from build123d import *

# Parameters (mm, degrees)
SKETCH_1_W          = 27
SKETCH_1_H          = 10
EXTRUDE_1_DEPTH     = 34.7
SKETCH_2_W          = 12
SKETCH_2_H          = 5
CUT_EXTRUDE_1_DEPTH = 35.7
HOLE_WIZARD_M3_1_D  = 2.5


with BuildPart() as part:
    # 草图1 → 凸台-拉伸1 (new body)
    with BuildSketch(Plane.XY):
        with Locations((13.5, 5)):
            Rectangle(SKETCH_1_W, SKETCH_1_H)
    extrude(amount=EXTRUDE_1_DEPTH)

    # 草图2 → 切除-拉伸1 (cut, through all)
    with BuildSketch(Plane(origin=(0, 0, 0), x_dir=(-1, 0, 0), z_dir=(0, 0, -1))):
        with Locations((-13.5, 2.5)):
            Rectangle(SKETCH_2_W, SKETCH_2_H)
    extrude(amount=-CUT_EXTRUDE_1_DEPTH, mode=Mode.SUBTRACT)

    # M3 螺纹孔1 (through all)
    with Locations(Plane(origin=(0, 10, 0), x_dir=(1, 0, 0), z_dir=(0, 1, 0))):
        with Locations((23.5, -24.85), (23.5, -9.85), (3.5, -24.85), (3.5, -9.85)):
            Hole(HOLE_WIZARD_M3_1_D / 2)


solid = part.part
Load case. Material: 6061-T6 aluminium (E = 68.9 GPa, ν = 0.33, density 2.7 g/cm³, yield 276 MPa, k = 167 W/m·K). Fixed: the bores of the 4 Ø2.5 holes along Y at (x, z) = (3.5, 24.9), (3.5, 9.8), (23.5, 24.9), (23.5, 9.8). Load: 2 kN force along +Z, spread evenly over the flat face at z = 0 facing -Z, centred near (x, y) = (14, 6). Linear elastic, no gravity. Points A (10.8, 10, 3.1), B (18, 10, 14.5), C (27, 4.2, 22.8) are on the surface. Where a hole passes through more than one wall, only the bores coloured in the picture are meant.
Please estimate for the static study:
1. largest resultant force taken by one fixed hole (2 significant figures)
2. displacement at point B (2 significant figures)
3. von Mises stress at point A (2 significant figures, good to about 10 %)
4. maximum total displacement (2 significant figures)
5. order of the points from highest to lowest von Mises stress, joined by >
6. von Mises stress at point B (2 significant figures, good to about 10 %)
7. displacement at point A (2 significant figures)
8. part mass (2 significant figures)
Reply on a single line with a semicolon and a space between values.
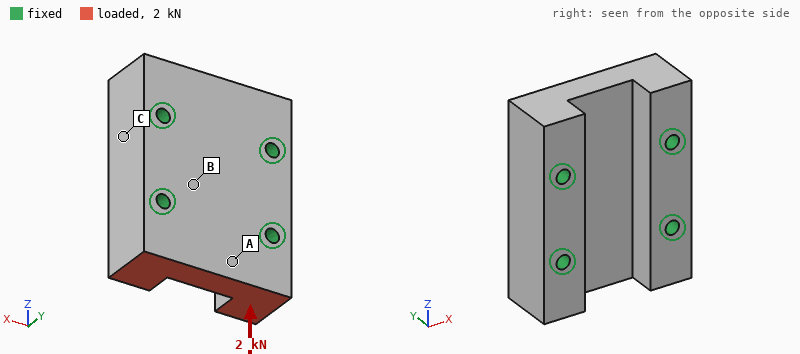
860 N; 0.58 µm; 8.2 MPa; 2.2 µm; A > B > C; 5.1 MPa; 1.8 µm; 19 g
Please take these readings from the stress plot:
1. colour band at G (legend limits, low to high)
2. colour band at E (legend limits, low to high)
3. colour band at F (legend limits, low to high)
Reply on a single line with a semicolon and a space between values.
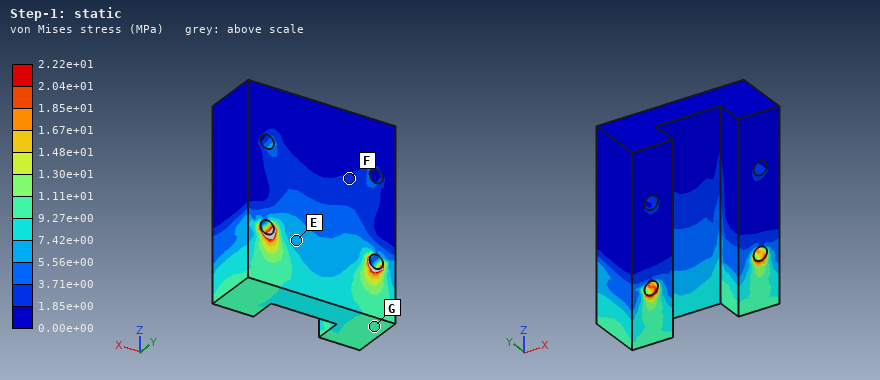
9.27e+00 to 1.11e+01 MPa; 5.56e+00 to 7.42e+00 MPa; 1.85e+00 to 3.71e+00 MPa
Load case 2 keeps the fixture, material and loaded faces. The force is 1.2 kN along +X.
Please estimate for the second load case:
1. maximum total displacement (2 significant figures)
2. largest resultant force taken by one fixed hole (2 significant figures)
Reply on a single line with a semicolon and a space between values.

6.6 µm; 750 N
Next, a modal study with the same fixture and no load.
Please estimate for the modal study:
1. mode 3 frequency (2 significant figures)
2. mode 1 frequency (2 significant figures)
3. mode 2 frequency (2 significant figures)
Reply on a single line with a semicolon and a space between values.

53 kHz; 43 kHz; 44 kHz
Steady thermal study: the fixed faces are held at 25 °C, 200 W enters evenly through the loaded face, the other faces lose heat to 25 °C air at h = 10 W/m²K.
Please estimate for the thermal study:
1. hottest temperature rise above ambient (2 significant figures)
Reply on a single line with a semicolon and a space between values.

64 K
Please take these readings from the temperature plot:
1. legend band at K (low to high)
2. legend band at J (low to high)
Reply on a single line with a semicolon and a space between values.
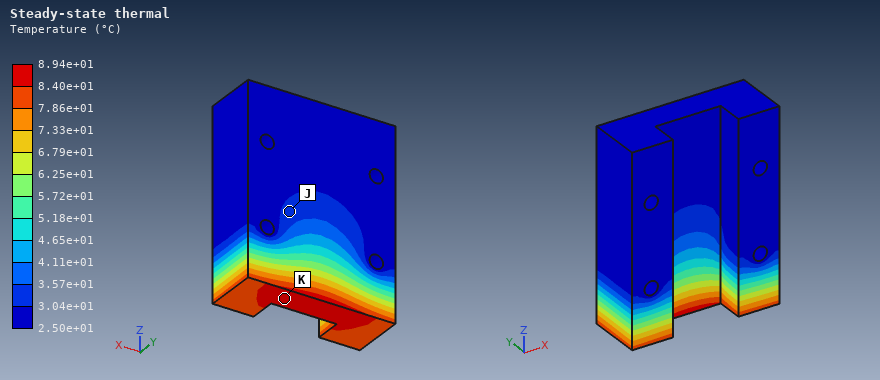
8.40e+01 to 8.94e+01 °C; 3.04e+01 to 3.57e+01 °C
